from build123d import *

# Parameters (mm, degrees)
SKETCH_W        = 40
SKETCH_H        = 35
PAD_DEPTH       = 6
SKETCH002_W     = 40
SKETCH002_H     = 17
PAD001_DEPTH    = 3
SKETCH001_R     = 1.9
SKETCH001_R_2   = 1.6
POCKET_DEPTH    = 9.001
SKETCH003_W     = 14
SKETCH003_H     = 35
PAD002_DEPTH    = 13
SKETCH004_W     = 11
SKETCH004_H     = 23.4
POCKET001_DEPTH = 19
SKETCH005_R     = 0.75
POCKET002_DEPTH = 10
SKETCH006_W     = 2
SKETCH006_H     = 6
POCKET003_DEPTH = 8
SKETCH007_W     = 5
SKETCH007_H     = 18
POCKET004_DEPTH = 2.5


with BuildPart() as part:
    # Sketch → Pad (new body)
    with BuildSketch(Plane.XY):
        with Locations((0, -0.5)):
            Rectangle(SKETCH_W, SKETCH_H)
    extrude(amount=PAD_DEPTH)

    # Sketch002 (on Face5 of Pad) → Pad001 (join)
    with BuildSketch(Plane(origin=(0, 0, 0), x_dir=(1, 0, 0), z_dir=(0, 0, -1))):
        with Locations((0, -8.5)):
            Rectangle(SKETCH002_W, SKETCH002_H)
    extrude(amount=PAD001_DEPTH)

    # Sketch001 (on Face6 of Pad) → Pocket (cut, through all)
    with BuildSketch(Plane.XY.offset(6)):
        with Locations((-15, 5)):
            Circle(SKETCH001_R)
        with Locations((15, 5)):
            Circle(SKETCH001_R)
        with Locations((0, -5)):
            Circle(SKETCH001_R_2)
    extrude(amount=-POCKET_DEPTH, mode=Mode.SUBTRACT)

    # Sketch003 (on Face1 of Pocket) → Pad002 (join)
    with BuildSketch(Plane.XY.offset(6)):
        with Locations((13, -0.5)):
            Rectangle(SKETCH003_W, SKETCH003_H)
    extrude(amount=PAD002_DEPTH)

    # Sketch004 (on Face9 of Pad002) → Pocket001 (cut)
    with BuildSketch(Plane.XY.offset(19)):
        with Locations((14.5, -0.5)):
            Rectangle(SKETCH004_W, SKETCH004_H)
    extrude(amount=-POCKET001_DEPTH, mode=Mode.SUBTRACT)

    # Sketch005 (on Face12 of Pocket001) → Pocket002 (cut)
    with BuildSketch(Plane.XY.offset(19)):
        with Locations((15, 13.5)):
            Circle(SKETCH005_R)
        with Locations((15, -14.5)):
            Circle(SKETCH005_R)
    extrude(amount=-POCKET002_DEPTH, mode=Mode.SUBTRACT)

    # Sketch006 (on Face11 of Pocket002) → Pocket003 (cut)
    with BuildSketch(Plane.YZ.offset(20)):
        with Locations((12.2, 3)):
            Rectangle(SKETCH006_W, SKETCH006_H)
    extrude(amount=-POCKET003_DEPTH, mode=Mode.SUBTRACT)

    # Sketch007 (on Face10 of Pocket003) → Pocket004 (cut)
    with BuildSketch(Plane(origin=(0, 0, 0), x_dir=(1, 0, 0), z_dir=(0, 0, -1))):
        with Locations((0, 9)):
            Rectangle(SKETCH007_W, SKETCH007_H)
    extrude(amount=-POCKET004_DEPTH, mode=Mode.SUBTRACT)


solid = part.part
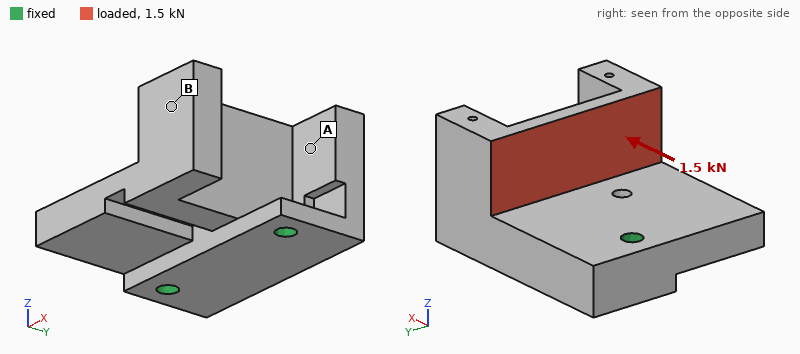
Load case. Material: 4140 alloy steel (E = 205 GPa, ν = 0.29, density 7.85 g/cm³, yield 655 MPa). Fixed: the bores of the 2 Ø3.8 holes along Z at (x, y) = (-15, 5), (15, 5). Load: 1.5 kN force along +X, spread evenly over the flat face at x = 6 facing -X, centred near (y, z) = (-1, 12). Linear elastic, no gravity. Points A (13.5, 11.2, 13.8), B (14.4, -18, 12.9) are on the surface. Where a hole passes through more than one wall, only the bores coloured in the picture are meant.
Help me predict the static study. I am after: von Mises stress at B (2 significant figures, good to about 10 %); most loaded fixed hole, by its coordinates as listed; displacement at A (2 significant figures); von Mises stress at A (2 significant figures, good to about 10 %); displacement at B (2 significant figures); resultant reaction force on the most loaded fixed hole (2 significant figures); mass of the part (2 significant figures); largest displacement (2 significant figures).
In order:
7.9 MPa
(-15, 5)
9.5 µm
23 MPa
32 µm
1.6 kN
89 g
49 µm
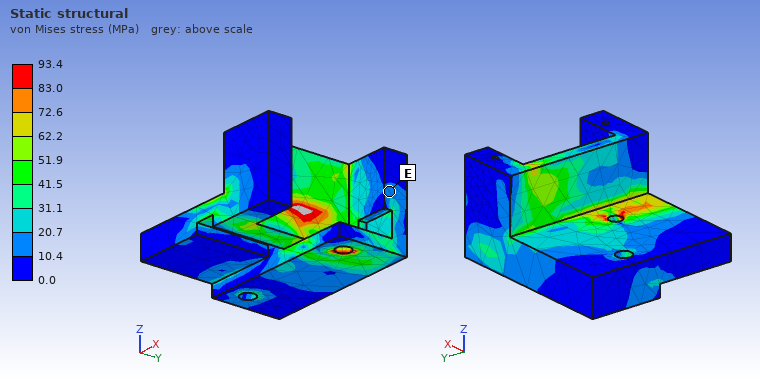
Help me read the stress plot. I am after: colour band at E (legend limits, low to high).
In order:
10.4 to 20.7 MPa
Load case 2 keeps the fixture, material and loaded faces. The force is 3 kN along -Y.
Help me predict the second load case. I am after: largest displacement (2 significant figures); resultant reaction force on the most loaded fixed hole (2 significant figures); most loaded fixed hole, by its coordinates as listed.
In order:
0.11 mm
1.8 kN
(15, 5)
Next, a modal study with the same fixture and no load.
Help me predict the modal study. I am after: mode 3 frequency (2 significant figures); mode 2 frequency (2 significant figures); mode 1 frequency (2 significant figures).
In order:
11 kHz
6800 Hz
4300 Hz
